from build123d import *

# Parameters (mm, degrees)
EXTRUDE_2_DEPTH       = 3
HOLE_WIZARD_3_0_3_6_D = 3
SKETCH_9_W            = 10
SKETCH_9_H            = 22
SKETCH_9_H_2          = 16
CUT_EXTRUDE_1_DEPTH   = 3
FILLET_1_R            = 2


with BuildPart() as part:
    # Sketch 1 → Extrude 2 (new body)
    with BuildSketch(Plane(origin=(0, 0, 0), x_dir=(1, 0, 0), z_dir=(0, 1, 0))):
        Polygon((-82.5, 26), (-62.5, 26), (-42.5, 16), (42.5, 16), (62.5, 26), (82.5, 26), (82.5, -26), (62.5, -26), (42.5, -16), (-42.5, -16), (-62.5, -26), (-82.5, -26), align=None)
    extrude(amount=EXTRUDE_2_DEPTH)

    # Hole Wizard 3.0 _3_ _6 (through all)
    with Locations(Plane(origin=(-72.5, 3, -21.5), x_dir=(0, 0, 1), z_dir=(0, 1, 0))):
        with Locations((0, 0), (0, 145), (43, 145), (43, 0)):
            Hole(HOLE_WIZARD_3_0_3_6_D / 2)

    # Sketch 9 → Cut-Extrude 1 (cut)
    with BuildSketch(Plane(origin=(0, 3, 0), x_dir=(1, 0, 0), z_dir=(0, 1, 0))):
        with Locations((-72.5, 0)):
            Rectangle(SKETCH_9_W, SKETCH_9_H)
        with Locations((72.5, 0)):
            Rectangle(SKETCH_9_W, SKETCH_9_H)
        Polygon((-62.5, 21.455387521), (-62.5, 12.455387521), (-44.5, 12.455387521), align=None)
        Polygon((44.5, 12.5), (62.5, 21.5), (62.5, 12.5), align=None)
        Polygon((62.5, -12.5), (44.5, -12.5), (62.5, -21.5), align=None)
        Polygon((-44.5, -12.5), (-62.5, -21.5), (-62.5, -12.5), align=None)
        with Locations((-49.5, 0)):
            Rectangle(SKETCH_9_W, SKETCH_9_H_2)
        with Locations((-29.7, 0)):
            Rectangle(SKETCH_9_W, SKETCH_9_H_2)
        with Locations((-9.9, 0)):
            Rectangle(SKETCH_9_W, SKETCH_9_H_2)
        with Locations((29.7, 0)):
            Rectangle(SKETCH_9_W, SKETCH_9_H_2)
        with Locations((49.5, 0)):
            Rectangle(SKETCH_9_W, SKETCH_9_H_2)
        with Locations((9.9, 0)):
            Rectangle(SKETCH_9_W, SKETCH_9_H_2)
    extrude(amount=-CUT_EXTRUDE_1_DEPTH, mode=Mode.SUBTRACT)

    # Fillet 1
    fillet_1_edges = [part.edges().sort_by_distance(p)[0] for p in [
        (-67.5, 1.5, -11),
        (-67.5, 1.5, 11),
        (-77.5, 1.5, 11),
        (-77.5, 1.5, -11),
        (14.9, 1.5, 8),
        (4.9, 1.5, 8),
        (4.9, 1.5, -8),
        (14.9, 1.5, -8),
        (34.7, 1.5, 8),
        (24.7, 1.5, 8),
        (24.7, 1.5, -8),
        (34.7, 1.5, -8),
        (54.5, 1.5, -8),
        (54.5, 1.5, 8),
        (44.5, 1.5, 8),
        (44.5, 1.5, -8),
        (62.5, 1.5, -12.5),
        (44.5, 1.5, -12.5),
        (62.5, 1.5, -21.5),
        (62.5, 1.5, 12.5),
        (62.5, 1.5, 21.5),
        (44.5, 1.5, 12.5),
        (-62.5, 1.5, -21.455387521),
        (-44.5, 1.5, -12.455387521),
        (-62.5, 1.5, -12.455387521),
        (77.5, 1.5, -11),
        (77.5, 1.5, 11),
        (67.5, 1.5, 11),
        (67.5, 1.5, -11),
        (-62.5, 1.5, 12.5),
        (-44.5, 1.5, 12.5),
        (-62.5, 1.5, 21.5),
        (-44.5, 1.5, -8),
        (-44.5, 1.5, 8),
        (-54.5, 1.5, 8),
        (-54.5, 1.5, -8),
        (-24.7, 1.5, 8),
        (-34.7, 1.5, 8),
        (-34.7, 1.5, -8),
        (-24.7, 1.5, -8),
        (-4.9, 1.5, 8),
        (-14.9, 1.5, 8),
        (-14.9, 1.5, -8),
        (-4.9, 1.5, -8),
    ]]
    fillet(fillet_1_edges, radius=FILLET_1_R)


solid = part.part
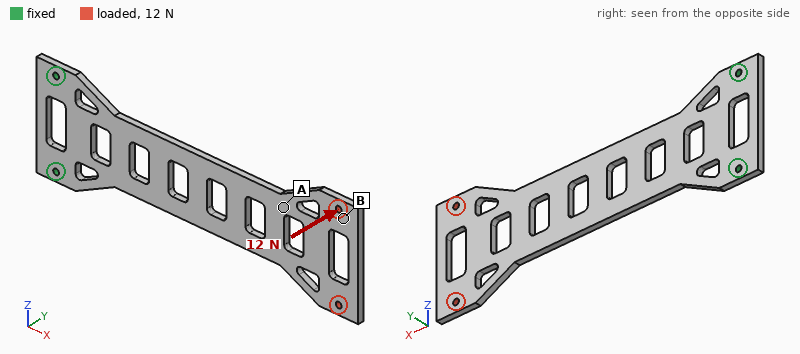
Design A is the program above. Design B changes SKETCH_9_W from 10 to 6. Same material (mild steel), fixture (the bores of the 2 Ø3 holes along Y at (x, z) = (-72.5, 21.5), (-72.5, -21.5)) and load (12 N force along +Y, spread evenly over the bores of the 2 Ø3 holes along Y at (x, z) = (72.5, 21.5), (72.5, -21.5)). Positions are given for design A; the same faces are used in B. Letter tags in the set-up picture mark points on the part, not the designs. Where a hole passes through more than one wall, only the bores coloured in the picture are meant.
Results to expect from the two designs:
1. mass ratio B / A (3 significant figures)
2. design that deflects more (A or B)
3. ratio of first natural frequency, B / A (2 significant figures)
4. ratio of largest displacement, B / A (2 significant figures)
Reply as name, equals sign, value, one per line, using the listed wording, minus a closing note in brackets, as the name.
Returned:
mass ratio B / A = 1.12
design that deflects more = A
ratio of first natural frequency, B / A = 0.99
ratio of largest displacement, B / A = 0.91
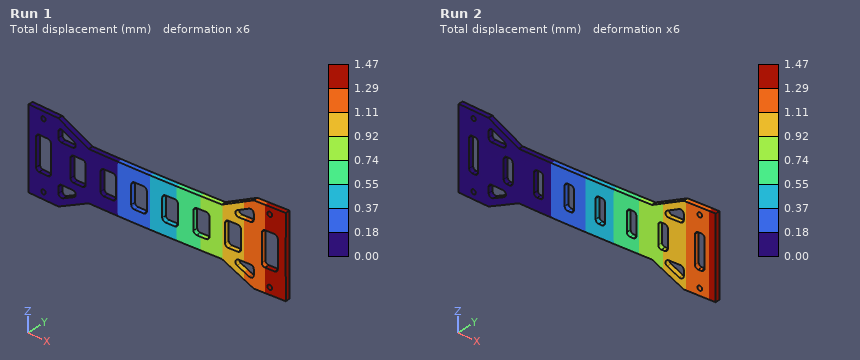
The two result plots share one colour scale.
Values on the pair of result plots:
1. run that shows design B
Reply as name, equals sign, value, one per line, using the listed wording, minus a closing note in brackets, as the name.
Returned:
run that shows design B = Run 2
